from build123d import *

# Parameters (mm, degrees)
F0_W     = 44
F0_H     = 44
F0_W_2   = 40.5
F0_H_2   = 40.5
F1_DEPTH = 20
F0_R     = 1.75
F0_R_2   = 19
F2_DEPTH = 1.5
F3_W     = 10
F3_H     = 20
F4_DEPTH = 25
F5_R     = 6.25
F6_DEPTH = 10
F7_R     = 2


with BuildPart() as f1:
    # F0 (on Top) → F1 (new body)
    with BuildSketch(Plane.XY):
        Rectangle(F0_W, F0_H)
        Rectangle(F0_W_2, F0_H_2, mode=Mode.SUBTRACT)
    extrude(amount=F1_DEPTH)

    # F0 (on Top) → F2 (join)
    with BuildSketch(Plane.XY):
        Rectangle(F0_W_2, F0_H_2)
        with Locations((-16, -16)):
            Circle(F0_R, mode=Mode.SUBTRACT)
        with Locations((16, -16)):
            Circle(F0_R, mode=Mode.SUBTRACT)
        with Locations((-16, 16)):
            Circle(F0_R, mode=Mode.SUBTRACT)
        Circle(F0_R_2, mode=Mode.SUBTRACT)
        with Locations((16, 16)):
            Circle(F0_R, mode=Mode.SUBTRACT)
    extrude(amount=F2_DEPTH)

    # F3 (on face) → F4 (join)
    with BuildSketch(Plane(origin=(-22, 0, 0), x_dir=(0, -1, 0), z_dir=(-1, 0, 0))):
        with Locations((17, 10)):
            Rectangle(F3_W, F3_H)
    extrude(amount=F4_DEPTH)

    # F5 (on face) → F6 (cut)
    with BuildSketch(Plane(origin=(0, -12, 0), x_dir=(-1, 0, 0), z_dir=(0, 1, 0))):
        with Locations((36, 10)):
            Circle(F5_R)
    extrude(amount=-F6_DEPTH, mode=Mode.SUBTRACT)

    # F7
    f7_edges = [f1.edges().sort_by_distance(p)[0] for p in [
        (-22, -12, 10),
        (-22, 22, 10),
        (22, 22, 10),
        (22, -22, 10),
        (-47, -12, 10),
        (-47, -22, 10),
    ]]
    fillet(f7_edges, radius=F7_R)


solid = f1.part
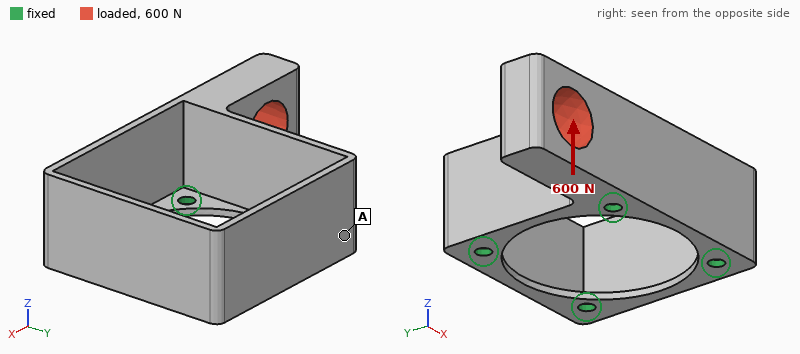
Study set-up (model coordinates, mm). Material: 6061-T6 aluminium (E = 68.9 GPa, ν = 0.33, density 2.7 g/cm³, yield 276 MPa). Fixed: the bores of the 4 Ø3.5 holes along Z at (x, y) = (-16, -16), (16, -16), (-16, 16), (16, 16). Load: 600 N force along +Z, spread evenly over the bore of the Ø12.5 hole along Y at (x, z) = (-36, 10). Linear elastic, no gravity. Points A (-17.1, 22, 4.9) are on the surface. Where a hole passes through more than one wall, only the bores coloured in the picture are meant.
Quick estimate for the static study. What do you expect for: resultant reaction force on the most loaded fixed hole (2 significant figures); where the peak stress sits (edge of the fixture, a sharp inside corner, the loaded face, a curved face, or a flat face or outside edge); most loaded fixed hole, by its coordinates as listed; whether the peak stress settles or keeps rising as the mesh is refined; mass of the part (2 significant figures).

960 N
edge of the fixture
(-16, -16)
keeps rising
28 g
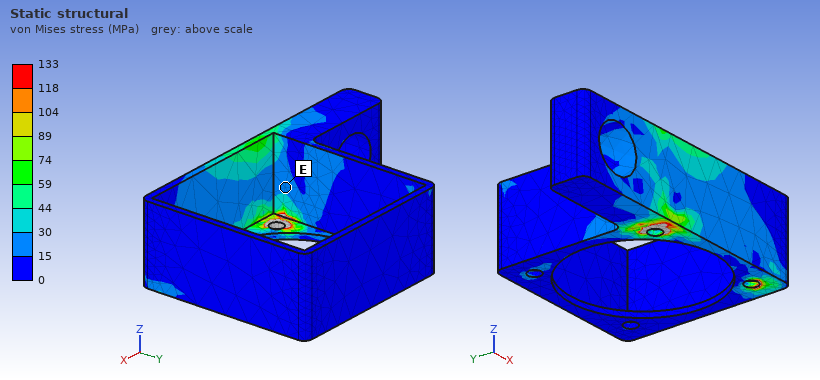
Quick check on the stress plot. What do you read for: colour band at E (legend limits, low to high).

15 to 30 MPa
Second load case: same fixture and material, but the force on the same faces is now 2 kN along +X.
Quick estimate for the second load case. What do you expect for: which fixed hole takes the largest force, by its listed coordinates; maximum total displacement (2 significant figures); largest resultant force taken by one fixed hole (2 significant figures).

(-16, -16)
0.18 mm
1.5 kN
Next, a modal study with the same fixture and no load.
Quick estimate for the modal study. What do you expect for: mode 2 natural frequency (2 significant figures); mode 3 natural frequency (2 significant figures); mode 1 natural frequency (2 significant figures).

4500 Hz
4900 Hz
3100 Hz
